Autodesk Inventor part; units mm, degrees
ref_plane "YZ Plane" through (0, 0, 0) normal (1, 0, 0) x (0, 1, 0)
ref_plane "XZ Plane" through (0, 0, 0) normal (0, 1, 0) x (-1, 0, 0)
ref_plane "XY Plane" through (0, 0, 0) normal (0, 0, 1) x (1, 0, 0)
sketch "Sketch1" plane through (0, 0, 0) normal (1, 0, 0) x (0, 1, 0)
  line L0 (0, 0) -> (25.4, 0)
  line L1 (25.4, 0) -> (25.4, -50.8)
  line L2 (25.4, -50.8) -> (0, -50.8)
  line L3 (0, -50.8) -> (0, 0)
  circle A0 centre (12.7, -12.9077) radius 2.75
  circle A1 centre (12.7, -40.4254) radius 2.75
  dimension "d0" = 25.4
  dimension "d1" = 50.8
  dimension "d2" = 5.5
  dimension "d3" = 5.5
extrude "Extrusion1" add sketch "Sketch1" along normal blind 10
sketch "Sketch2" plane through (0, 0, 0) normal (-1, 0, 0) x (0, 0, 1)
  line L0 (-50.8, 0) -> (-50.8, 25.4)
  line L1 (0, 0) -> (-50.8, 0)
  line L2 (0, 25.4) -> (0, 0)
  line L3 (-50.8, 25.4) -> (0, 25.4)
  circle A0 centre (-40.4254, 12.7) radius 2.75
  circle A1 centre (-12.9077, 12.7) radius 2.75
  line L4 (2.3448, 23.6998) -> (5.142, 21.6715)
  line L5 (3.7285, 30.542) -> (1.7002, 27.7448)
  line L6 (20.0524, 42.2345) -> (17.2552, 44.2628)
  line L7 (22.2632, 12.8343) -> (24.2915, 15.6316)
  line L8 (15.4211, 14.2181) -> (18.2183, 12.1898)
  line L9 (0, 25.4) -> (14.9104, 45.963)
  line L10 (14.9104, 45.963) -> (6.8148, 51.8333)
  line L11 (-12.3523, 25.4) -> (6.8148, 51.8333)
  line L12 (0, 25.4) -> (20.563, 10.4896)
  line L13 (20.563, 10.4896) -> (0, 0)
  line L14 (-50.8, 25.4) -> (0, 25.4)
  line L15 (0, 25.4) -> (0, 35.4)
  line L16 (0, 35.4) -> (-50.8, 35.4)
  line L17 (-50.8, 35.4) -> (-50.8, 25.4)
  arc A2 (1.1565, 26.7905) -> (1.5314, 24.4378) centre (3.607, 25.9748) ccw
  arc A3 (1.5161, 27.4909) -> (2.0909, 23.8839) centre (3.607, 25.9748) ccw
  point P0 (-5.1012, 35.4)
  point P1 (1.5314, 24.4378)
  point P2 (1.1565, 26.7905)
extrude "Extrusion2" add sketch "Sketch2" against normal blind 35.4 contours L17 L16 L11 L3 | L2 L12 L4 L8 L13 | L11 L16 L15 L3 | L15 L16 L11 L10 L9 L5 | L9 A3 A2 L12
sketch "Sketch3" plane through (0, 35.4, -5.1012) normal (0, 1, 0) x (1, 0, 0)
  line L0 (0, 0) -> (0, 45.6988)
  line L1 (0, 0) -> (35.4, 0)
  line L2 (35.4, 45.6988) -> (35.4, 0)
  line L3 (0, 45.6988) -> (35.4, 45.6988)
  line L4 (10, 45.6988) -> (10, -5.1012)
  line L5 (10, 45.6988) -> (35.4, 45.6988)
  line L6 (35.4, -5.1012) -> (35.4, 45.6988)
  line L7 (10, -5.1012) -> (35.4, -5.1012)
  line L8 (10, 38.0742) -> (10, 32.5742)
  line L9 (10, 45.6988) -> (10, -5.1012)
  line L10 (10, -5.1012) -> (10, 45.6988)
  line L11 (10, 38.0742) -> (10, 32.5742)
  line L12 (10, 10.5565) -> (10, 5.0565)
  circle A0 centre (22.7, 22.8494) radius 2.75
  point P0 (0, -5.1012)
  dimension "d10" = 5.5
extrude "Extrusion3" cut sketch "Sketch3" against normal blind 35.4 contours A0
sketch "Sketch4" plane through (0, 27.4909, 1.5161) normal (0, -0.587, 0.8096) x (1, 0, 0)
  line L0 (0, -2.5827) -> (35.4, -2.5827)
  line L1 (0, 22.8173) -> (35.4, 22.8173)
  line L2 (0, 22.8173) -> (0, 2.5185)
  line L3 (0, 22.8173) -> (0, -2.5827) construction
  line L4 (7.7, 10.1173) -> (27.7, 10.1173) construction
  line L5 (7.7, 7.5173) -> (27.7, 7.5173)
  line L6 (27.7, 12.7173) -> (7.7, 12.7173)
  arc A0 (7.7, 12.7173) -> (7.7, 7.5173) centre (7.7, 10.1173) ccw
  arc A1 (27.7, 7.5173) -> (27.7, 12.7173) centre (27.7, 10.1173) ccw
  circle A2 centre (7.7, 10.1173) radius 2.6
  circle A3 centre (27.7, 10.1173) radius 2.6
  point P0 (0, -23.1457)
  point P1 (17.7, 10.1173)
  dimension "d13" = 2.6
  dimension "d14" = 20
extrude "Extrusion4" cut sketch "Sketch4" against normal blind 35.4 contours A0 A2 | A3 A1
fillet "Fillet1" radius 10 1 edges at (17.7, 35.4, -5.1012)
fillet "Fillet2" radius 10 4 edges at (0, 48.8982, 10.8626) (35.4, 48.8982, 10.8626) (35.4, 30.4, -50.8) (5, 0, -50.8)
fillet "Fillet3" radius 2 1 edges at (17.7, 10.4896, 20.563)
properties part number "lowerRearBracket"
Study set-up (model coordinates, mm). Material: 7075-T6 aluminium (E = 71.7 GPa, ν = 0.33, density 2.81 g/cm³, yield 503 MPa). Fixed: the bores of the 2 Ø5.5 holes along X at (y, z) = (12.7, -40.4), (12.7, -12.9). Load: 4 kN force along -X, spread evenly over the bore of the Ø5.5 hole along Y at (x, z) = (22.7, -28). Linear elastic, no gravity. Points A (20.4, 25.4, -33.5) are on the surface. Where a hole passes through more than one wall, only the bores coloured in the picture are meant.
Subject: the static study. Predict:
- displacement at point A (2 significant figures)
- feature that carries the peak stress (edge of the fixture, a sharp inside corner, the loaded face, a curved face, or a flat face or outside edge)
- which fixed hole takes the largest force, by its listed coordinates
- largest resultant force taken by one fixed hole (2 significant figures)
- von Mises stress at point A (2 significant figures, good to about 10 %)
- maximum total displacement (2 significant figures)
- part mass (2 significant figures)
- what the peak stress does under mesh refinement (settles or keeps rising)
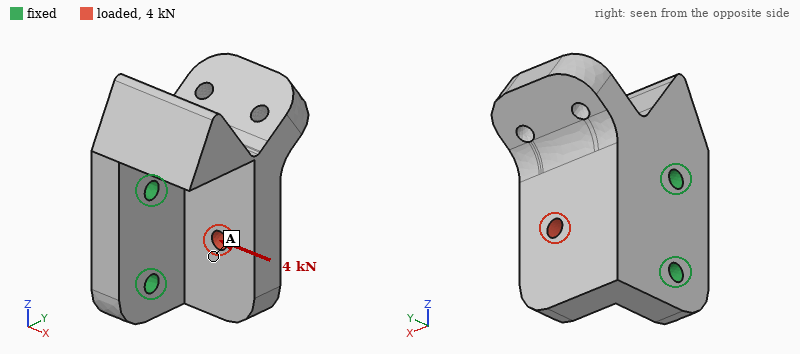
40 µm
edge of the fixture
(12.7, -40.4)
2.1 kN
20 MPa
77 µm
130 g
keeps rising
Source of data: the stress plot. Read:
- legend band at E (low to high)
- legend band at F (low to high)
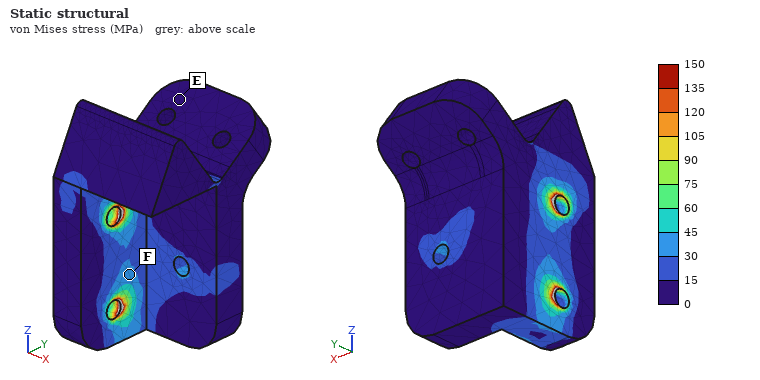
0 to 15 MPa
30 to 45 MPa
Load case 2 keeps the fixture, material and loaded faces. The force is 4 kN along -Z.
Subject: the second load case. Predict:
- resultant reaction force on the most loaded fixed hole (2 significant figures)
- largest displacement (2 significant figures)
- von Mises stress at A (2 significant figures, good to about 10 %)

3.6 kN
60 µm
29 MPa
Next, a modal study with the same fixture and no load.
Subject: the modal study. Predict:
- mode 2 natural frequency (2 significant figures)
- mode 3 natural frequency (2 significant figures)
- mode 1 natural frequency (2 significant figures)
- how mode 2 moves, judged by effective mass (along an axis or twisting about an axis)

5300 Hz
7000 Hz
3400 Hz
along Z
